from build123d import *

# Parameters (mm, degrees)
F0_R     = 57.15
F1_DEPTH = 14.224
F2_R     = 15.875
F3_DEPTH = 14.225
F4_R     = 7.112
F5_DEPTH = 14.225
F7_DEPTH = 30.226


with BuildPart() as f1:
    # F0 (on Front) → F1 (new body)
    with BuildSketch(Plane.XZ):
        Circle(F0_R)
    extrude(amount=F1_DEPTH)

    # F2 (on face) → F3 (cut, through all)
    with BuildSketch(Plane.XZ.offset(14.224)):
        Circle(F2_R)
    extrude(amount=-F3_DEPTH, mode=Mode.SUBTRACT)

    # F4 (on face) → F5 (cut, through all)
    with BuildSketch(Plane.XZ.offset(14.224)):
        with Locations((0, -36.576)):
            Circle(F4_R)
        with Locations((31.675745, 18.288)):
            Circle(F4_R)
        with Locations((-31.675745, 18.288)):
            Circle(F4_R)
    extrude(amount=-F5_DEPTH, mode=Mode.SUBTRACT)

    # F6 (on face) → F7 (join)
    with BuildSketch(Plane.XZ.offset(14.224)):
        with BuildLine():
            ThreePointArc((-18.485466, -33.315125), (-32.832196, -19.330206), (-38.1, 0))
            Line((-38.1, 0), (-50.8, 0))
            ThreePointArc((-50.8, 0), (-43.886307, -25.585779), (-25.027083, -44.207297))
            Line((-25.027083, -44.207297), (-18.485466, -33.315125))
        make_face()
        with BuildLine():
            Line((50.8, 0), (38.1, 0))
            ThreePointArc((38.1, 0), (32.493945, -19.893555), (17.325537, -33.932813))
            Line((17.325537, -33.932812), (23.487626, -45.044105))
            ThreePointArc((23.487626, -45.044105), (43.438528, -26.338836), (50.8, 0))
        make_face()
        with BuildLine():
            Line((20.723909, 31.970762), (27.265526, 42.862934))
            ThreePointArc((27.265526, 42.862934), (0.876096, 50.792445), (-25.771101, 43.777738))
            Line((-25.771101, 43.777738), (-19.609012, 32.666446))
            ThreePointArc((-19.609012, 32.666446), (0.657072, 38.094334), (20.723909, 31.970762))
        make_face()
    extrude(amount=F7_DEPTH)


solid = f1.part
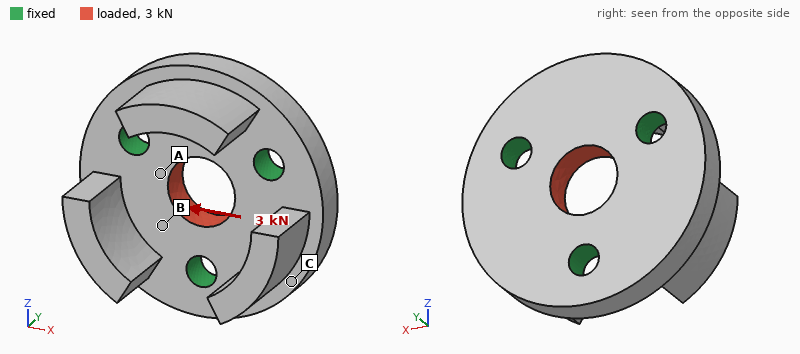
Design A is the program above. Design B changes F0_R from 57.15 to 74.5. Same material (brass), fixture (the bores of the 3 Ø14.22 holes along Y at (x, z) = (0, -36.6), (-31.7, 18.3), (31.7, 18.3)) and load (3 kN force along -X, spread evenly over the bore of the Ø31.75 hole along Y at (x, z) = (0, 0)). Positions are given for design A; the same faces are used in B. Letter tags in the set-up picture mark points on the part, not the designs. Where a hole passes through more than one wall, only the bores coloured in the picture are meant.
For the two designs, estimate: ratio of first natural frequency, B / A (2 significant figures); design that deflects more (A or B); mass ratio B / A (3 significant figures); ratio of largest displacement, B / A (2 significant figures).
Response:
0.79
A
1.56
0.92
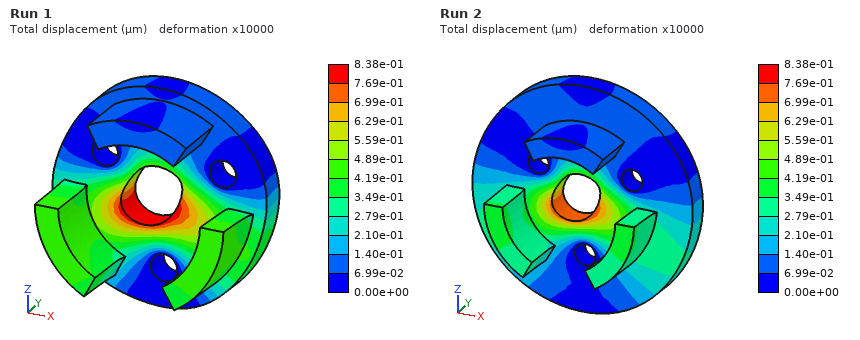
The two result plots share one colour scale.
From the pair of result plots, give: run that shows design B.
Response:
Run 2
